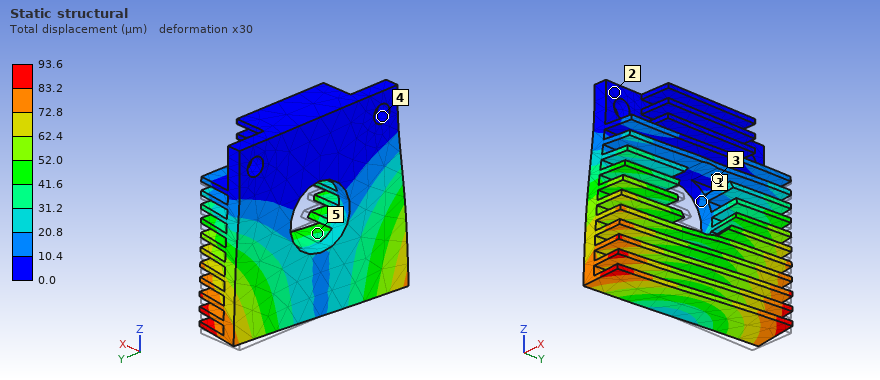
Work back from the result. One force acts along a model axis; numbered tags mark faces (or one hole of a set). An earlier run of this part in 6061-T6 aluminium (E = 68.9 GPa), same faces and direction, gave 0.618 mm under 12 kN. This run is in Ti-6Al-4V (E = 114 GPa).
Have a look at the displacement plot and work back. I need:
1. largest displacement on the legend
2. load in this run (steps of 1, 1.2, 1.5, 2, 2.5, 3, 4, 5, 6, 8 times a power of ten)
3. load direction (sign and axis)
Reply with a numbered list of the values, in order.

1. 93.6 µm
2. 3 kN
3. -Y
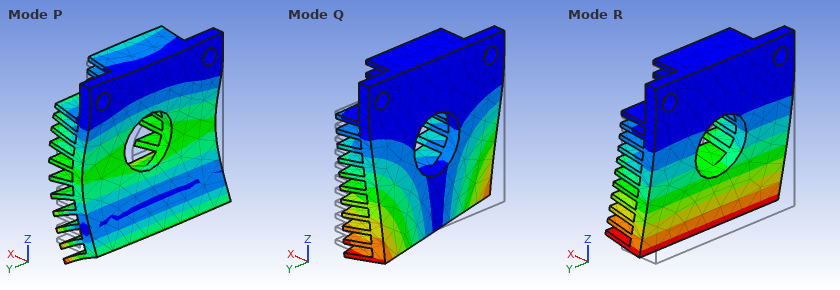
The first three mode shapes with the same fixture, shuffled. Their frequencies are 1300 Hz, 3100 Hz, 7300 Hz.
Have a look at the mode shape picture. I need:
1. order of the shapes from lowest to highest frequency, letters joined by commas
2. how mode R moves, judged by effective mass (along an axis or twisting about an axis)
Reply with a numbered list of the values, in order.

1. R, Q, P
2. along X
